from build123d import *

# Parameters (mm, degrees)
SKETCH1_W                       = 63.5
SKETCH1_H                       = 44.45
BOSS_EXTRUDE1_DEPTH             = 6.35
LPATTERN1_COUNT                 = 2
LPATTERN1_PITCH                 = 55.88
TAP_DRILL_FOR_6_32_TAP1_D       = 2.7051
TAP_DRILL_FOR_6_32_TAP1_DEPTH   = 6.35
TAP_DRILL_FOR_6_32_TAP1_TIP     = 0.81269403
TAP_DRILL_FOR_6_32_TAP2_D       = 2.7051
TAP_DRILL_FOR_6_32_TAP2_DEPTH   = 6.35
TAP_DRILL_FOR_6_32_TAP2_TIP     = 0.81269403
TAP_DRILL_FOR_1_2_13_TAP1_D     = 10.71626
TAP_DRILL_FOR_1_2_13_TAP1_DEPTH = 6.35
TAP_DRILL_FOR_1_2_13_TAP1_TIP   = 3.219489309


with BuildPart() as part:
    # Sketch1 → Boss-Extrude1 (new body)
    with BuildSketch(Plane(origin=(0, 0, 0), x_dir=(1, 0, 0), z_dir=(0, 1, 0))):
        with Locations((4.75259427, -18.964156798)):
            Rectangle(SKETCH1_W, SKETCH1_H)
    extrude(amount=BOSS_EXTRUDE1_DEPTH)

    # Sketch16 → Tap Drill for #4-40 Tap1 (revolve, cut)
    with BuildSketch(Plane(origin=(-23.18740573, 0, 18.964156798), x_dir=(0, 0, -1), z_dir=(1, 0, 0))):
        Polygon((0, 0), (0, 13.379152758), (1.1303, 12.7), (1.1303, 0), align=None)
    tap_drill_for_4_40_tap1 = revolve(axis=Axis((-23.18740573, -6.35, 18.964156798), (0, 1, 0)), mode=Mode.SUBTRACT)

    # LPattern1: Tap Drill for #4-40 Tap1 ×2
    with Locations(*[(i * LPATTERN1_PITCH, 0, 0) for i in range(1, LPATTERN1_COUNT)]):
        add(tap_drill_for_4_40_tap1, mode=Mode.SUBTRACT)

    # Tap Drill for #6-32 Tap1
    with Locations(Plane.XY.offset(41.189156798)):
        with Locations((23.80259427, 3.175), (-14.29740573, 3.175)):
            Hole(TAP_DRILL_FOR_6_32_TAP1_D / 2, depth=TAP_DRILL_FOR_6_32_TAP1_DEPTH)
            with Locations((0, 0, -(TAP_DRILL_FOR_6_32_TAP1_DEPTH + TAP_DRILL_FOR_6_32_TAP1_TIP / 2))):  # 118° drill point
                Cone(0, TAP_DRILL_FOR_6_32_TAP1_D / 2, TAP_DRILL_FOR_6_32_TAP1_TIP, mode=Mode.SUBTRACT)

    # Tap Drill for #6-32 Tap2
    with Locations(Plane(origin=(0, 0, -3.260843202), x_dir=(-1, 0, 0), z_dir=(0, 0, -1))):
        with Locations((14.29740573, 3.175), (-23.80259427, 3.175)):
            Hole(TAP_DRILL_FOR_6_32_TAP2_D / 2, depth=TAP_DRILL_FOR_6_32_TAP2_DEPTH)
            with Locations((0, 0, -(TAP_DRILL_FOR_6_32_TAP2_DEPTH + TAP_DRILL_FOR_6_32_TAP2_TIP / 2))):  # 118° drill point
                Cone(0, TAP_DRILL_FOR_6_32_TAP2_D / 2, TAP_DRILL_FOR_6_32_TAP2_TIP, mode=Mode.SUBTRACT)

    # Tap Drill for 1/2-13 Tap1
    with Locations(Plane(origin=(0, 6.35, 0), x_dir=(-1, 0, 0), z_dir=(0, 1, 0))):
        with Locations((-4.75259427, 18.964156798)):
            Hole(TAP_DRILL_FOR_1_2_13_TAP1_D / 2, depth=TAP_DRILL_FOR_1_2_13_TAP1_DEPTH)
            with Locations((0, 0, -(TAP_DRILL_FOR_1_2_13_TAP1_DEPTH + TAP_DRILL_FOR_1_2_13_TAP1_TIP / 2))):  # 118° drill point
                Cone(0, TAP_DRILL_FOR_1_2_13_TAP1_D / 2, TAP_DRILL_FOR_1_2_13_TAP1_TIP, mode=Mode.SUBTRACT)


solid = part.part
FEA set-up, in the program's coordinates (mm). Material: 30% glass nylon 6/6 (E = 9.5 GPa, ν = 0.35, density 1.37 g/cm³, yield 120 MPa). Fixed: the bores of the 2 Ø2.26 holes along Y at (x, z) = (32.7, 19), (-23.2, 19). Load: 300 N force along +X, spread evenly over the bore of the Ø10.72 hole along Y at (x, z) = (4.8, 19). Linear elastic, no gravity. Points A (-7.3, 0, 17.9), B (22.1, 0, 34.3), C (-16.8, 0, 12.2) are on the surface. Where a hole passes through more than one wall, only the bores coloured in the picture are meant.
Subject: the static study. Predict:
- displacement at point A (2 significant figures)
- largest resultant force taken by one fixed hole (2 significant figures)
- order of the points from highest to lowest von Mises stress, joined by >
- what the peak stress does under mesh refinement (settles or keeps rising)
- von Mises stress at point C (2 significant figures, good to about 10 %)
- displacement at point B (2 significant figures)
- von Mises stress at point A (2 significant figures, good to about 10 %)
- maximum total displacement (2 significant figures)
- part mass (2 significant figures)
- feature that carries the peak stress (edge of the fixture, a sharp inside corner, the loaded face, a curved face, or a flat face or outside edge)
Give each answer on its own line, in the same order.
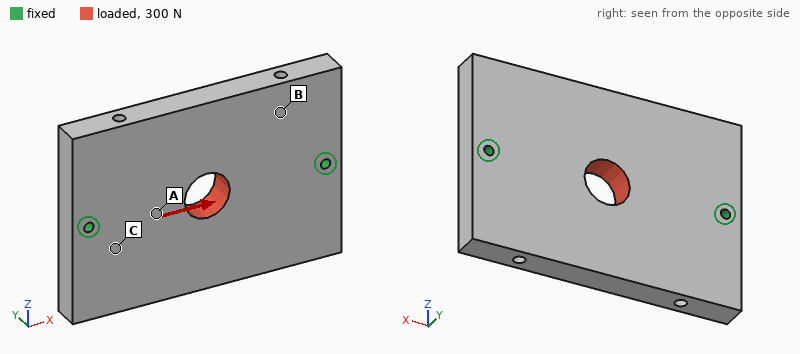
3.3 µm
150 N
A > C > B
keeps rising
0.94 MPa
3.0 µm
1.5 MPa
4.7 µm
23 g
edge of the fixture
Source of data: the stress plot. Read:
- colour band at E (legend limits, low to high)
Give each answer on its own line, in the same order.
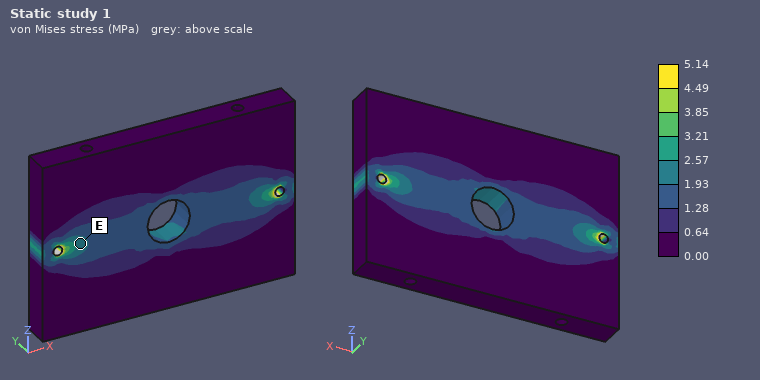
1.93 to 2.57 MPa
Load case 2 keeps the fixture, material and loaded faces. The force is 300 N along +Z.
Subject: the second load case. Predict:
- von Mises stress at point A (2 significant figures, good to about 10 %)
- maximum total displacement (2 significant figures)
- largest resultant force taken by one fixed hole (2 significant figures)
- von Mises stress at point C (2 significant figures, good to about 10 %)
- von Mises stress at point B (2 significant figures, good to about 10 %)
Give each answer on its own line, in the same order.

1.1 MPa
8.4 µm
150 N
1.4 MPa
0.99 MPa
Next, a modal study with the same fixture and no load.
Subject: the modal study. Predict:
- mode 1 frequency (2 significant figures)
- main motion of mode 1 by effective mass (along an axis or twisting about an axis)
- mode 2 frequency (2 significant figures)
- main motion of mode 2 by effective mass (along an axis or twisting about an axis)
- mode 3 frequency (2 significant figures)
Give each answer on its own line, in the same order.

2400 Hz
twisting about X
3100 Hz
along Y
5100 Hz
